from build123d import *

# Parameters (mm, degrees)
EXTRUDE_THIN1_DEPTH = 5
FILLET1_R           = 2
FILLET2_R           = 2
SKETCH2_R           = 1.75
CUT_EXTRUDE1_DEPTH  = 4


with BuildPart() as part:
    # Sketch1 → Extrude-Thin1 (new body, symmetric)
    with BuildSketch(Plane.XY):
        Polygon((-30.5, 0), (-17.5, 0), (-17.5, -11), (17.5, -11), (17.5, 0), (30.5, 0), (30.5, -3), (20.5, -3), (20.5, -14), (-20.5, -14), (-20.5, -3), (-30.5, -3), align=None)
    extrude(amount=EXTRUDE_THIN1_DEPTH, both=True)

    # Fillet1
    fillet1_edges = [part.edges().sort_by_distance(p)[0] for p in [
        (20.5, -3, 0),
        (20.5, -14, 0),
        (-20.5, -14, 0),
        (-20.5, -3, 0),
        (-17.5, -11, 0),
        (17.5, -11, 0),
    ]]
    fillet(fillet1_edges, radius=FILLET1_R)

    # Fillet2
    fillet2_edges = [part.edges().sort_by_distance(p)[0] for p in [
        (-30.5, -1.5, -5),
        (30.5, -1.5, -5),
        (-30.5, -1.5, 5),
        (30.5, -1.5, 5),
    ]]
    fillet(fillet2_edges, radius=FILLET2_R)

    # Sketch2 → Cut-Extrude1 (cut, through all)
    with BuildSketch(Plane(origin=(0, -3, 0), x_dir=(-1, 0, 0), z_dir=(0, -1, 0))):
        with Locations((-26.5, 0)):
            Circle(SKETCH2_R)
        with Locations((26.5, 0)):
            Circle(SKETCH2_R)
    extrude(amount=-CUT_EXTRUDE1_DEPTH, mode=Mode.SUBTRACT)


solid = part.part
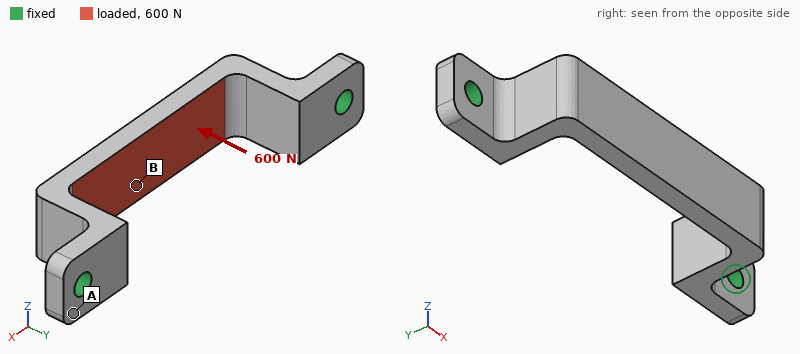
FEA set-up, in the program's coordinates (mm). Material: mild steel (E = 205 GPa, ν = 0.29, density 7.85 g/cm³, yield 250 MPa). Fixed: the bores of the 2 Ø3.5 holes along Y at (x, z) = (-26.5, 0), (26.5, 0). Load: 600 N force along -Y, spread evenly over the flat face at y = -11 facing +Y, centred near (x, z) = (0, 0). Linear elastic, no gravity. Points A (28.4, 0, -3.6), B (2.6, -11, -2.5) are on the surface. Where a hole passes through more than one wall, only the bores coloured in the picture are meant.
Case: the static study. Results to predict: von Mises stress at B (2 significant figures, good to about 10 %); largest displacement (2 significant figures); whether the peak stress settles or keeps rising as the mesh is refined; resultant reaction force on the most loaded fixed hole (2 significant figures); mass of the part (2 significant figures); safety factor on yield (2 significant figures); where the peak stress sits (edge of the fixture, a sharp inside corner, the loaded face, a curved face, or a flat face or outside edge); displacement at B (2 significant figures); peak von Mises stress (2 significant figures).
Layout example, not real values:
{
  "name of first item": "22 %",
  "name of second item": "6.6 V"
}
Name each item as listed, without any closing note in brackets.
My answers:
{
  "von Mises stress at B": "63 MPa",
  "largest displacement": "28 µm",
  "whether the peak stress settles or keeps rising as the mesh is refined": "settles",
  "resultant reaction force on the most loaded fixed hole": "430 N",
  "mass of the part": "19 g",
  "safety factor on yield": "1.9",
  "where the peak stress sits": "a curved face",
  "displacement at B": "26 µm",
  "peak von Mises stress": "130 MPa"
}
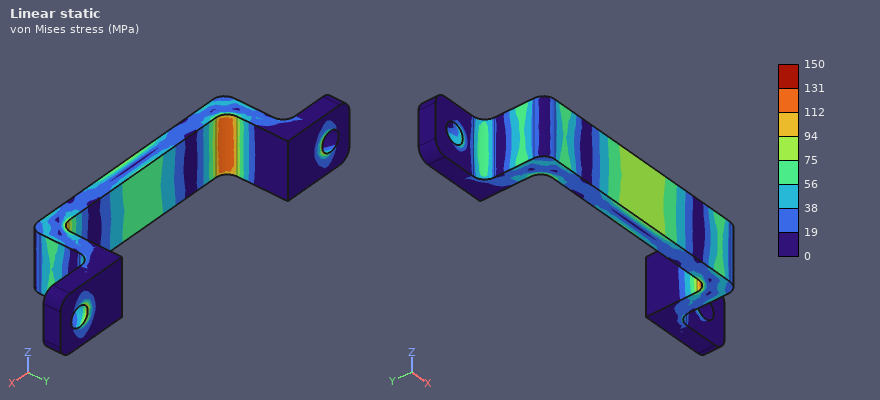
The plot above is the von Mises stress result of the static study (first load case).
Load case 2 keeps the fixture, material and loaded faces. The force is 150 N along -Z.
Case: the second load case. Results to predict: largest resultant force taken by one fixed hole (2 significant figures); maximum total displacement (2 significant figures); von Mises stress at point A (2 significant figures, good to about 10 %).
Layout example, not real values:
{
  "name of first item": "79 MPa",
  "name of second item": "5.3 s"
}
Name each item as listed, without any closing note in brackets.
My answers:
{
  "largest resultant force taken by one fixed hole": "75 N",
  "maximum total displacement": "9.4 µm",
  "von Mises stress at point A": "13 MPa"
}
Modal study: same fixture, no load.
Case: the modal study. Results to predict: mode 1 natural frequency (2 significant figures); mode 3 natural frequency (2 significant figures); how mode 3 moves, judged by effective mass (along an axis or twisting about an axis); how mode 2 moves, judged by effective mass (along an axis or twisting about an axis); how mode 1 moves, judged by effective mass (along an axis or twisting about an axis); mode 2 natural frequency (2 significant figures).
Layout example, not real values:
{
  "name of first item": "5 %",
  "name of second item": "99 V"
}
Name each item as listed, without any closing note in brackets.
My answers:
{
  "mode 1 natural frequency": "6300 Hz",
  "mode 3 natural frequency": "9800 Hz",
  "how mode 3 moves, judged by effective mass": "along Y",
  "how mode 2 moves, judged by effective mass": "along X",
  "how mode 1 moves, judged by effective mass": "along Z",
  "mode 2 natural frequency": "7600 Hz"
}
